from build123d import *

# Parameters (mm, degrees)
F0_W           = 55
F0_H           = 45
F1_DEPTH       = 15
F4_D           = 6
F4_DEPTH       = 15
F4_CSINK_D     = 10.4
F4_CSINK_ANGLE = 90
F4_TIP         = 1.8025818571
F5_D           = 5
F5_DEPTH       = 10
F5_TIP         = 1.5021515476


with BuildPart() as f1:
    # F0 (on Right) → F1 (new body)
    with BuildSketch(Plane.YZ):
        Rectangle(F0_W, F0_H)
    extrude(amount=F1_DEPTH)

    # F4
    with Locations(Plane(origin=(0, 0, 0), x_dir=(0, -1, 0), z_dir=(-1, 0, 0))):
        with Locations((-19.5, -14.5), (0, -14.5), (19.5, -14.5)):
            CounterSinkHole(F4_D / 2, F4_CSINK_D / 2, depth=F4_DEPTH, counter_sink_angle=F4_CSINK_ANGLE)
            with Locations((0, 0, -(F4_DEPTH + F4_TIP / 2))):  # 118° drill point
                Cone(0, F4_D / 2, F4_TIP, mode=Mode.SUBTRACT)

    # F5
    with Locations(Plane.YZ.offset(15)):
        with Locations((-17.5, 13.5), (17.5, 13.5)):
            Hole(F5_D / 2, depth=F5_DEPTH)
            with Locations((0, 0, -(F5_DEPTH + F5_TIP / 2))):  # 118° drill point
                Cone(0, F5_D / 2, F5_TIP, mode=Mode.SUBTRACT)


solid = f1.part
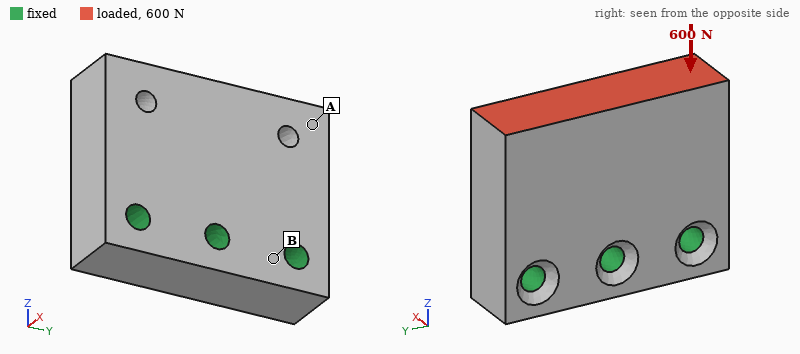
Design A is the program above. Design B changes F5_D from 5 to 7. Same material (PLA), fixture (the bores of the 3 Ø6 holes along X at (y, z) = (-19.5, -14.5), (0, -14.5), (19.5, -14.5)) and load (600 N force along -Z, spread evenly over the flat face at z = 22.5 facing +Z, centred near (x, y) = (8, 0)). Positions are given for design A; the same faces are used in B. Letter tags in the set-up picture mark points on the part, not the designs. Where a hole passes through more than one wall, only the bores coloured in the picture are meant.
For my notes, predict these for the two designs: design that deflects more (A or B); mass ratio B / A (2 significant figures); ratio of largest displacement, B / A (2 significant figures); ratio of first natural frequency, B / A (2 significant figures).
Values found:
B
0.99
1.1
1.0
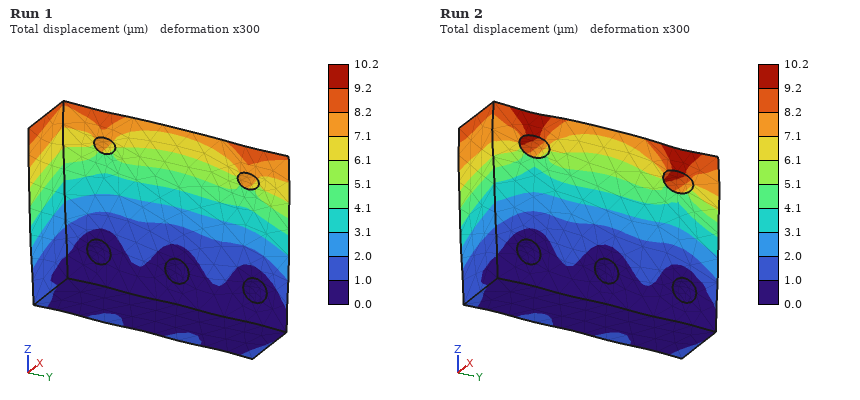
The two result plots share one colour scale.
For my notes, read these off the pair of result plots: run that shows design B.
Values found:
Run 2
